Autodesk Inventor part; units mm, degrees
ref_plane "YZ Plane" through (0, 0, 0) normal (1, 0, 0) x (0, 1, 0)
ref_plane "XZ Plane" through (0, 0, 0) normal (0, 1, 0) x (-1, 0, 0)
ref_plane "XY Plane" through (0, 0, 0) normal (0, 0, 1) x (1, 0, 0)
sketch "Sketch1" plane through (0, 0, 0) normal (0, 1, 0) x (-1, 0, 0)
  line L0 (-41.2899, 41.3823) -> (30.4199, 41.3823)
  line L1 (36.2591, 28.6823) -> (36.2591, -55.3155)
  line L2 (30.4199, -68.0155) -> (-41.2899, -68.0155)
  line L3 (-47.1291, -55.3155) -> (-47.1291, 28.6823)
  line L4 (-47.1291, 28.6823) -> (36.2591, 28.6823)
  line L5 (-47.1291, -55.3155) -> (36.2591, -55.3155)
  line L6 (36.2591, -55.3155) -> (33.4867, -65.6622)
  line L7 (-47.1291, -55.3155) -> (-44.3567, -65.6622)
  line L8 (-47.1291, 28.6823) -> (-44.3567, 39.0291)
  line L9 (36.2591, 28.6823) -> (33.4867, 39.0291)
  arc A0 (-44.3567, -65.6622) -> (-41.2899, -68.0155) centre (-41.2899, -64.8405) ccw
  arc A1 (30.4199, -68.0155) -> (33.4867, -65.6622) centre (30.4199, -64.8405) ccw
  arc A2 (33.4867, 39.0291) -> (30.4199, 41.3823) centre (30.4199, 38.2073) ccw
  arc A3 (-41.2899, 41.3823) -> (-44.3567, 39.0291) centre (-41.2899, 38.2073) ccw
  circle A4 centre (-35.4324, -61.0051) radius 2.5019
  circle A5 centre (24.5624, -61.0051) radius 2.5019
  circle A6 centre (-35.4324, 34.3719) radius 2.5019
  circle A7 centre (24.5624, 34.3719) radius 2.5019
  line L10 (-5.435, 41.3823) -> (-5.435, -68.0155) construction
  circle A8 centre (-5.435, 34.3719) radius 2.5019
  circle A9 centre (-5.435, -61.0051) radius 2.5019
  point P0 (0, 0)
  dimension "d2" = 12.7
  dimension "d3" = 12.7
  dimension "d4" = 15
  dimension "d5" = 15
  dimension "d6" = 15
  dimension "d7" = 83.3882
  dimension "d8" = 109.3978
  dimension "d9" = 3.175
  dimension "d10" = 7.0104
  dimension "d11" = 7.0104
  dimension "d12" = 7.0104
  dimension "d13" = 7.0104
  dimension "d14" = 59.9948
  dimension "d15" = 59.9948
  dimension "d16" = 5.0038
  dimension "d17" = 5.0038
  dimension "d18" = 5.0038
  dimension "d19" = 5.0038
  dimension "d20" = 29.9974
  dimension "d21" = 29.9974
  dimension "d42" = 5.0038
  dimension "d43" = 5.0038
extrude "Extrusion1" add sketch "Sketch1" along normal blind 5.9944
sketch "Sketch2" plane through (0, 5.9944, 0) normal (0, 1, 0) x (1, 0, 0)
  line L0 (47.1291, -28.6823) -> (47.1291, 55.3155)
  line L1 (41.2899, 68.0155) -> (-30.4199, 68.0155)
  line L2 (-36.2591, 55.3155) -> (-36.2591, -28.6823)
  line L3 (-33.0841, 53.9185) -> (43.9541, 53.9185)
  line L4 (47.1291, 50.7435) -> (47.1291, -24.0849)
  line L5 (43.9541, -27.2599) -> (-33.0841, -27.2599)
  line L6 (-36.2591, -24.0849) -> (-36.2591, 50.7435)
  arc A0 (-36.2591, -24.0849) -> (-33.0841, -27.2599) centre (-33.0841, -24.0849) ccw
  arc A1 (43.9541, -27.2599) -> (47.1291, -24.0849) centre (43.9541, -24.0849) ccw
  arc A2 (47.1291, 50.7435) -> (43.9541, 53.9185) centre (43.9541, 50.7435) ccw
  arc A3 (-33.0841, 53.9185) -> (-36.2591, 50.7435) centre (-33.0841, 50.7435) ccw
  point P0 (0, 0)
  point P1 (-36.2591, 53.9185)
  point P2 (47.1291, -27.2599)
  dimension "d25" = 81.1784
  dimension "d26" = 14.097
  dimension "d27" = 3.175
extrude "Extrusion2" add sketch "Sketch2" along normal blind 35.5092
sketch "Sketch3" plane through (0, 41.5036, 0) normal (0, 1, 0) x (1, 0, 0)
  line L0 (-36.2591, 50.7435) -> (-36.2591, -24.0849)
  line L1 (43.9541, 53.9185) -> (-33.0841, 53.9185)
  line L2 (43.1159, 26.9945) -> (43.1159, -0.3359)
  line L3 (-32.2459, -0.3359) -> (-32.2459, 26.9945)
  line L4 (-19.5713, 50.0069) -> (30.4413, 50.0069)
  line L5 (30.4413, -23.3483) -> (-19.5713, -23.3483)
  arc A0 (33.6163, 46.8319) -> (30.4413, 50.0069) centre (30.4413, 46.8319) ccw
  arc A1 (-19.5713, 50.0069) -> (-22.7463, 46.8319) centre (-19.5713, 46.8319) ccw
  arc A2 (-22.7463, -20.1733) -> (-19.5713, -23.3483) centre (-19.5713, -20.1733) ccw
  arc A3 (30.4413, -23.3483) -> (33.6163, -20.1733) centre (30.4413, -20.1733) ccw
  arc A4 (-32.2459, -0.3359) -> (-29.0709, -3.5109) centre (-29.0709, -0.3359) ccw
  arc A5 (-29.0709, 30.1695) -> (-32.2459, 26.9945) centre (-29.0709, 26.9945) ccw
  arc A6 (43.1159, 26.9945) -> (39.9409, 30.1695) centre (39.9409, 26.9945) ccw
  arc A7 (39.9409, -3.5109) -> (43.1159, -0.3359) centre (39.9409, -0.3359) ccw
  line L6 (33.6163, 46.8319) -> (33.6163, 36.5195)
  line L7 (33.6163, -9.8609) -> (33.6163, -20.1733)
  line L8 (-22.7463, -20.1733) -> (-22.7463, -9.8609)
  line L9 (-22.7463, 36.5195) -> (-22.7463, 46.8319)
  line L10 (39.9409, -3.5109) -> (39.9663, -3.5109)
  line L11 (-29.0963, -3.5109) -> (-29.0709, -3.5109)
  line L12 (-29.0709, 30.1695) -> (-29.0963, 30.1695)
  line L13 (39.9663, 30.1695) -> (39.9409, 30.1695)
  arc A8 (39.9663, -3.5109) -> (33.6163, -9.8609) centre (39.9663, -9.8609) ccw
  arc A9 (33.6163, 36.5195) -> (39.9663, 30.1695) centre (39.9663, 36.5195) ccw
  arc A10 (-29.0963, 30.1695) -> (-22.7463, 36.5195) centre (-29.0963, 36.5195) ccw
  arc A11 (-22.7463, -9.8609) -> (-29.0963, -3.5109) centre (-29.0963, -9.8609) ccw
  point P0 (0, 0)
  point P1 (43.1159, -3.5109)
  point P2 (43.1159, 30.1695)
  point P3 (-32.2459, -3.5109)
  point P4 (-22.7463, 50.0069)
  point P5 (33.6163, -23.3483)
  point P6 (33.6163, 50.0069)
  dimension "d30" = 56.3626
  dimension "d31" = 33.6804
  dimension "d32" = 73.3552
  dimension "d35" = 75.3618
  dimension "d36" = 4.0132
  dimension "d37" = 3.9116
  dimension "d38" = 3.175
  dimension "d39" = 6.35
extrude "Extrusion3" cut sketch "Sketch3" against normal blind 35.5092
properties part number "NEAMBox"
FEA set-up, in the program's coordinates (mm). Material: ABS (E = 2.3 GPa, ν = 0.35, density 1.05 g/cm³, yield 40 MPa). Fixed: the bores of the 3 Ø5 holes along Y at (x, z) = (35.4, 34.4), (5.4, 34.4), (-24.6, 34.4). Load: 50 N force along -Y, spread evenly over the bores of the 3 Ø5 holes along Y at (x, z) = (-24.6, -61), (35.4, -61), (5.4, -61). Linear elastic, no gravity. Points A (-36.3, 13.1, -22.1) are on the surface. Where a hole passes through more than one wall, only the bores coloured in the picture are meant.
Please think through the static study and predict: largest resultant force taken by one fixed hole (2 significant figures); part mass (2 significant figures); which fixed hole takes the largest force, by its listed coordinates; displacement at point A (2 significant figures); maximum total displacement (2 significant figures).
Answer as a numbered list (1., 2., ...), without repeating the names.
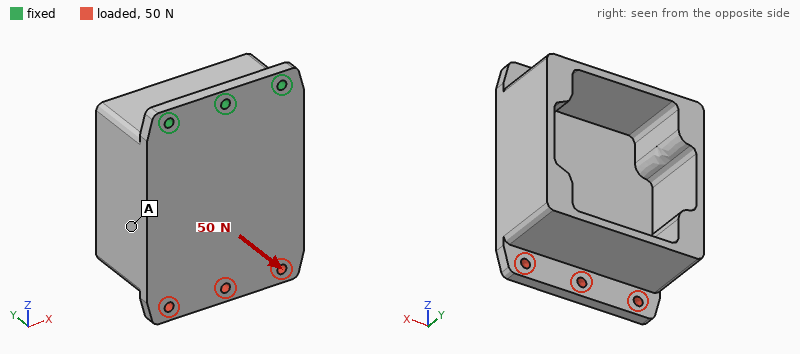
1. 46 N
2. 130 g
3. (5.4, 34.4)
4. 0.90 mm
5. 1.7 mm
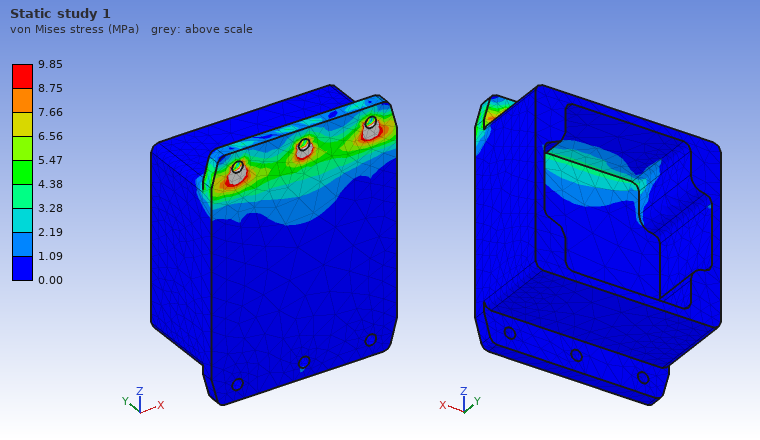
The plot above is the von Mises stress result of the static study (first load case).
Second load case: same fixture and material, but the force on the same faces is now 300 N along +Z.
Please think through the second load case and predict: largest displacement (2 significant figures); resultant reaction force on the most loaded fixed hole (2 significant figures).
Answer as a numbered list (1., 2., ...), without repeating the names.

1. 59 µm
2. 100 N
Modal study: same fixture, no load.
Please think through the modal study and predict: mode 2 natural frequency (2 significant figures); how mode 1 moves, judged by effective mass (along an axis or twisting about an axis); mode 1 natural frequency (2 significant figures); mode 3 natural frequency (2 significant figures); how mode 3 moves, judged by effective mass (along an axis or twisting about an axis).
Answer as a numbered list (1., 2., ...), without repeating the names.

1. 330 Hz
2. along Y
3. 130 Hz
4. 860 Hz
5. along X
